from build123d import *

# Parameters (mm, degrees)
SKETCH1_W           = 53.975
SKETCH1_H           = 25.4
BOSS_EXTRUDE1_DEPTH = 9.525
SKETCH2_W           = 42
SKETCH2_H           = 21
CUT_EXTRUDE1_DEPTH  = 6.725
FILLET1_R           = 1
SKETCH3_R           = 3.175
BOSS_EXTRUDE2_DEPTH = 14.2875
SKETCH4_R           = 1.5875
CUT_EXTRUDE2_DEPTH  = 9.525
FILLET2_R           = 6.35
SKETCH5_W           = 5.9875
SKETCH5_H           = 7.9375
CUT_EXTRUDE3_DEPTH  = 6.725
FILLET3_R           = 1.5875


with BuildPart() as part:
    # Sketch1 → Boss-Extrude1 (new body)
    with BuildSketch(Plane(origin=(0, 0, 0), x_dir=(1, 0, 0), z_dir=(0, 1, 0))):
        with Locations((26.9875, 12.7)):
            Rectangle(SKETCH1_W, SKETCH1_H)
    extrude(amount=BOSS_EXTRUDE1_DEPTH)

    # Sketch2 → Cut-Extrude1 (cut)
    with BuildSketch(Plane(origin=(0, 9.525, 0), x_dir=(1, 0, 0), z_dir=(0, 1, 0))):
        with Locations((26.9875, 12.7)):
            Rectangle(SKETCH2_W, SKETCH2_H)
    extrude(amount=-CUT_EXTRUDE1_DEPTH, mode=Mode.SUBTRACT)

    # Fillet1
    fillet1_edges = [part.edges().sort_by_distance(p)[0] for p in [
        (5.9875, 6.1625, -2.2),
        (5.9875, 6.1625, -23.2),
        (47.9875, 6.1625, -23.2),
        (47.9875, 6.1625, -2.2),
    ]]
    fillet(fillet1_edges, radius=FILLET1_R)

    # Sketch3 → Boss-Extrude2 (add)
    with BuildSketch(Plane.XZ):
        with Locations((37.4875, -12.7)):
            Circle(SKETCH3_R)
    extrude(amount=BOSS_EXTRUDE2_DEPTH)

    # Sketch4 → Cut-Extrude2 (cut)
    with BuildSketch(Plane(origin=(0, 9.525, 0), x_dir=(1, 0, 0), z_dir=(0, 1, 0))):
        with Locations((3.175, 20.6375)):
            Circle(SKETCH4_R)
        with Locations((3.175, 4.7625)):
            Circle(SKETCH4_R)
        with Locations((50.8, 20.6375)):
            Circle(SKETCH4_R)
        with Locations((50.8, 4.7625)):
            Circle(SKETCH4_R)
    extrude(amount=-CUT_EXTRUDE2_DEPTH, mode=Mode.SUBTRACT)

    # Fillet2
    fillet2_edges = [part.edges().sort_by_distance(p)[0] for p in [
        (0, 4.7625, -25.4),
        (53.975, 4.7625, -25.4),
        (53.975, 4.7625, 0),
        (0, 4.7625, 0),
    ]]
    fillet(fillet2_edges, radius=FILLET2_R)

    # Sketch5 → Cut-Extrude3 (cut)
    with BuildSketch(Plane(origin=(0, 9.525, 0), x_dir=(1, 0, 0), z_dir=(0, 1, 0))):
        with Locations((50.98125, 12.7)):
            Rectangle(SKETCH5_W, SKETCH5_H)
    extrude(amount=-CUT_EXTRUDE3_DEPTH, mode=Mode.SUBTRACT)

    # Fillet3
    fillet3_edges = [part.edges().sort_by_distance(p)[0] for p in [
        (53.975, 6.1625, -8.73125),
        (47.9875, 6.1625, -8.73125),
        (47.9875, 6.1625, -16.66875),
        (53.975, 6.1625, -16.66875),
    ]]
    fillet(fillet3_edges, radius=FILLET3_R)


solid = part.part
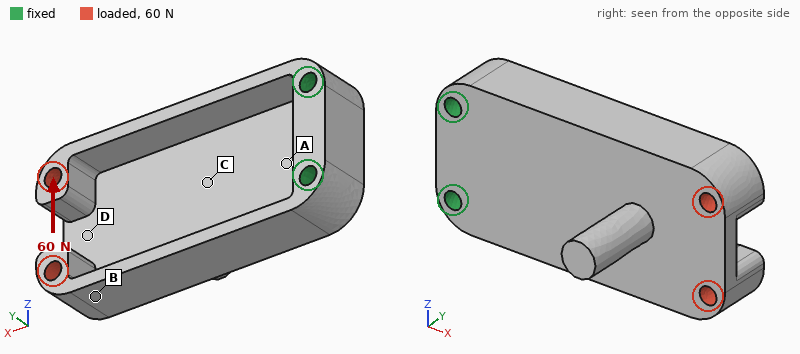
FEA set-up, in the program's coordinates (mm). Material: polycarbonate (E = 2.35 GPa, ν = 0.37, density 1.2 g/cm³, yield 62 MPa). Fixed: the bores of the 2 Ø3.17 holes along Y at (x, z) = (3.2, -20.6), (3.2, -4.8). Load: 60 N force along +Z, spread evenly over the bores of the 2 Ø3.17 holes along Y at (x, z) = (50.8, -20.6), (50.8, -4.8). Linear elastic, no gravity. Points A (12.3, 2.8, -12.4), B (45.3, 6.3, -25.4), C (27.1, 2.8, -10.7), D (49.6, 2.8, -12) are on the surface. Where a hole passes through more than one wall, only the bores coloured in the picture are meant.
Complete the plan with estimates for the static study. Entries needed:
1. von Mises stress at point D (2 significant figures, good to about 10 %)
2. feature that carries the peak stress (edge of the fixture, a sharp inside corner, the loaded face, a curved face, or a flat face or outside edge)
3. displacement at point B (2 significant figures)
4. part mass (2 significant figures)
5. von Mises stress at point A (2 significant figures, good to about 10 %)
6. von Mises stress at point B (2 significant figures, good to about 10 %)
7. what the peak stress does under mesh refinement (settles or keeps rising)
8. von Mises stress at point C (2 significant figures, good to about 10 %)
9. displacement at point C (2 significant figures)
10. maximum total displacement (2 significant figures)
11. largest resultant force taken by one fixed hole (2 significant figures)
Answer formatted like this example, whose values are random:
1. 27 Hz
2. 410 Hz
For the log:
1. 6.5 MPa
2. edge of the fixture
3. 0.52 mm
4. 7.9 g
5. 4.4 MPa
6. 2.9 MPa
7. keeps rising
8. 5.5 MPa
9. 0.12 mm
10. 0.66 mm
11. 160 N
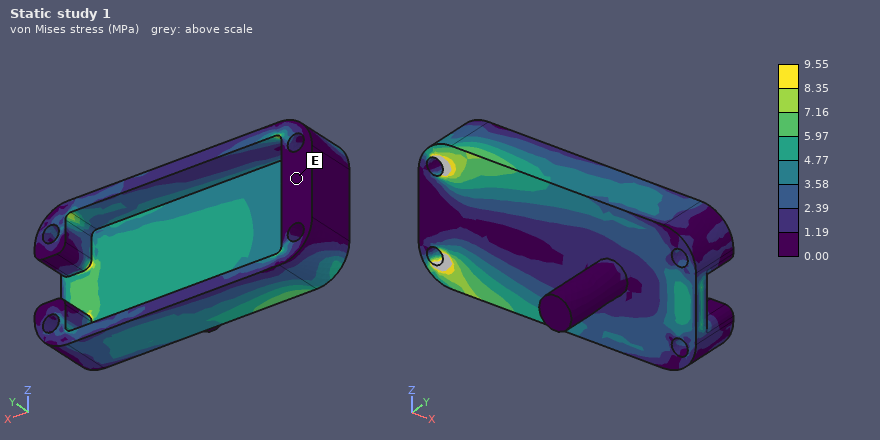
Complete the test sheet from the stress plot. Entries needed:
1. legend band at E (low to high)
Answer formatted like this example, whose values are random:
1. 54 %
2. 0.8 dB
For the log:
1. 0.00 to 1.19 MPa
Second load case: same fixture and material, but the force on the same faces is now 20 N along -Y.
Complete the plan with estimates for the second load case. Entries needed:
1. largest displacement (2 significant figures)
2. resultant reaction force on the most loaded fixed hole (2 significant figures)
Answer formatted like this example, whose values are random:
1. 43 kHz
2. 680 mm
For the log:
1. 0.65 mm
2. 15 N
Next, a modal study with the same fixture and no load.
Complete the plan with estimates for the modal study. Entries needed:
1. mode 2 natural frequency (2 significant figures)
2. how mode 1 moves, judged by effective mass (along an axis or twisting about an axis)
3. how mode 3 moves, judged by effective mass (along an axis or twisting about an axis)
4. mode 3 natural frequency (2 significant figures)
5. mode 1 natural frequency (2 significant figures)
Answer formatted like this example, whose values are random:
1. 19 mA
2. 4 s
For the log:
1. 1000 Hz
2. along Y
3. along Z
4. 1800 Hz
5. 610 Hz
